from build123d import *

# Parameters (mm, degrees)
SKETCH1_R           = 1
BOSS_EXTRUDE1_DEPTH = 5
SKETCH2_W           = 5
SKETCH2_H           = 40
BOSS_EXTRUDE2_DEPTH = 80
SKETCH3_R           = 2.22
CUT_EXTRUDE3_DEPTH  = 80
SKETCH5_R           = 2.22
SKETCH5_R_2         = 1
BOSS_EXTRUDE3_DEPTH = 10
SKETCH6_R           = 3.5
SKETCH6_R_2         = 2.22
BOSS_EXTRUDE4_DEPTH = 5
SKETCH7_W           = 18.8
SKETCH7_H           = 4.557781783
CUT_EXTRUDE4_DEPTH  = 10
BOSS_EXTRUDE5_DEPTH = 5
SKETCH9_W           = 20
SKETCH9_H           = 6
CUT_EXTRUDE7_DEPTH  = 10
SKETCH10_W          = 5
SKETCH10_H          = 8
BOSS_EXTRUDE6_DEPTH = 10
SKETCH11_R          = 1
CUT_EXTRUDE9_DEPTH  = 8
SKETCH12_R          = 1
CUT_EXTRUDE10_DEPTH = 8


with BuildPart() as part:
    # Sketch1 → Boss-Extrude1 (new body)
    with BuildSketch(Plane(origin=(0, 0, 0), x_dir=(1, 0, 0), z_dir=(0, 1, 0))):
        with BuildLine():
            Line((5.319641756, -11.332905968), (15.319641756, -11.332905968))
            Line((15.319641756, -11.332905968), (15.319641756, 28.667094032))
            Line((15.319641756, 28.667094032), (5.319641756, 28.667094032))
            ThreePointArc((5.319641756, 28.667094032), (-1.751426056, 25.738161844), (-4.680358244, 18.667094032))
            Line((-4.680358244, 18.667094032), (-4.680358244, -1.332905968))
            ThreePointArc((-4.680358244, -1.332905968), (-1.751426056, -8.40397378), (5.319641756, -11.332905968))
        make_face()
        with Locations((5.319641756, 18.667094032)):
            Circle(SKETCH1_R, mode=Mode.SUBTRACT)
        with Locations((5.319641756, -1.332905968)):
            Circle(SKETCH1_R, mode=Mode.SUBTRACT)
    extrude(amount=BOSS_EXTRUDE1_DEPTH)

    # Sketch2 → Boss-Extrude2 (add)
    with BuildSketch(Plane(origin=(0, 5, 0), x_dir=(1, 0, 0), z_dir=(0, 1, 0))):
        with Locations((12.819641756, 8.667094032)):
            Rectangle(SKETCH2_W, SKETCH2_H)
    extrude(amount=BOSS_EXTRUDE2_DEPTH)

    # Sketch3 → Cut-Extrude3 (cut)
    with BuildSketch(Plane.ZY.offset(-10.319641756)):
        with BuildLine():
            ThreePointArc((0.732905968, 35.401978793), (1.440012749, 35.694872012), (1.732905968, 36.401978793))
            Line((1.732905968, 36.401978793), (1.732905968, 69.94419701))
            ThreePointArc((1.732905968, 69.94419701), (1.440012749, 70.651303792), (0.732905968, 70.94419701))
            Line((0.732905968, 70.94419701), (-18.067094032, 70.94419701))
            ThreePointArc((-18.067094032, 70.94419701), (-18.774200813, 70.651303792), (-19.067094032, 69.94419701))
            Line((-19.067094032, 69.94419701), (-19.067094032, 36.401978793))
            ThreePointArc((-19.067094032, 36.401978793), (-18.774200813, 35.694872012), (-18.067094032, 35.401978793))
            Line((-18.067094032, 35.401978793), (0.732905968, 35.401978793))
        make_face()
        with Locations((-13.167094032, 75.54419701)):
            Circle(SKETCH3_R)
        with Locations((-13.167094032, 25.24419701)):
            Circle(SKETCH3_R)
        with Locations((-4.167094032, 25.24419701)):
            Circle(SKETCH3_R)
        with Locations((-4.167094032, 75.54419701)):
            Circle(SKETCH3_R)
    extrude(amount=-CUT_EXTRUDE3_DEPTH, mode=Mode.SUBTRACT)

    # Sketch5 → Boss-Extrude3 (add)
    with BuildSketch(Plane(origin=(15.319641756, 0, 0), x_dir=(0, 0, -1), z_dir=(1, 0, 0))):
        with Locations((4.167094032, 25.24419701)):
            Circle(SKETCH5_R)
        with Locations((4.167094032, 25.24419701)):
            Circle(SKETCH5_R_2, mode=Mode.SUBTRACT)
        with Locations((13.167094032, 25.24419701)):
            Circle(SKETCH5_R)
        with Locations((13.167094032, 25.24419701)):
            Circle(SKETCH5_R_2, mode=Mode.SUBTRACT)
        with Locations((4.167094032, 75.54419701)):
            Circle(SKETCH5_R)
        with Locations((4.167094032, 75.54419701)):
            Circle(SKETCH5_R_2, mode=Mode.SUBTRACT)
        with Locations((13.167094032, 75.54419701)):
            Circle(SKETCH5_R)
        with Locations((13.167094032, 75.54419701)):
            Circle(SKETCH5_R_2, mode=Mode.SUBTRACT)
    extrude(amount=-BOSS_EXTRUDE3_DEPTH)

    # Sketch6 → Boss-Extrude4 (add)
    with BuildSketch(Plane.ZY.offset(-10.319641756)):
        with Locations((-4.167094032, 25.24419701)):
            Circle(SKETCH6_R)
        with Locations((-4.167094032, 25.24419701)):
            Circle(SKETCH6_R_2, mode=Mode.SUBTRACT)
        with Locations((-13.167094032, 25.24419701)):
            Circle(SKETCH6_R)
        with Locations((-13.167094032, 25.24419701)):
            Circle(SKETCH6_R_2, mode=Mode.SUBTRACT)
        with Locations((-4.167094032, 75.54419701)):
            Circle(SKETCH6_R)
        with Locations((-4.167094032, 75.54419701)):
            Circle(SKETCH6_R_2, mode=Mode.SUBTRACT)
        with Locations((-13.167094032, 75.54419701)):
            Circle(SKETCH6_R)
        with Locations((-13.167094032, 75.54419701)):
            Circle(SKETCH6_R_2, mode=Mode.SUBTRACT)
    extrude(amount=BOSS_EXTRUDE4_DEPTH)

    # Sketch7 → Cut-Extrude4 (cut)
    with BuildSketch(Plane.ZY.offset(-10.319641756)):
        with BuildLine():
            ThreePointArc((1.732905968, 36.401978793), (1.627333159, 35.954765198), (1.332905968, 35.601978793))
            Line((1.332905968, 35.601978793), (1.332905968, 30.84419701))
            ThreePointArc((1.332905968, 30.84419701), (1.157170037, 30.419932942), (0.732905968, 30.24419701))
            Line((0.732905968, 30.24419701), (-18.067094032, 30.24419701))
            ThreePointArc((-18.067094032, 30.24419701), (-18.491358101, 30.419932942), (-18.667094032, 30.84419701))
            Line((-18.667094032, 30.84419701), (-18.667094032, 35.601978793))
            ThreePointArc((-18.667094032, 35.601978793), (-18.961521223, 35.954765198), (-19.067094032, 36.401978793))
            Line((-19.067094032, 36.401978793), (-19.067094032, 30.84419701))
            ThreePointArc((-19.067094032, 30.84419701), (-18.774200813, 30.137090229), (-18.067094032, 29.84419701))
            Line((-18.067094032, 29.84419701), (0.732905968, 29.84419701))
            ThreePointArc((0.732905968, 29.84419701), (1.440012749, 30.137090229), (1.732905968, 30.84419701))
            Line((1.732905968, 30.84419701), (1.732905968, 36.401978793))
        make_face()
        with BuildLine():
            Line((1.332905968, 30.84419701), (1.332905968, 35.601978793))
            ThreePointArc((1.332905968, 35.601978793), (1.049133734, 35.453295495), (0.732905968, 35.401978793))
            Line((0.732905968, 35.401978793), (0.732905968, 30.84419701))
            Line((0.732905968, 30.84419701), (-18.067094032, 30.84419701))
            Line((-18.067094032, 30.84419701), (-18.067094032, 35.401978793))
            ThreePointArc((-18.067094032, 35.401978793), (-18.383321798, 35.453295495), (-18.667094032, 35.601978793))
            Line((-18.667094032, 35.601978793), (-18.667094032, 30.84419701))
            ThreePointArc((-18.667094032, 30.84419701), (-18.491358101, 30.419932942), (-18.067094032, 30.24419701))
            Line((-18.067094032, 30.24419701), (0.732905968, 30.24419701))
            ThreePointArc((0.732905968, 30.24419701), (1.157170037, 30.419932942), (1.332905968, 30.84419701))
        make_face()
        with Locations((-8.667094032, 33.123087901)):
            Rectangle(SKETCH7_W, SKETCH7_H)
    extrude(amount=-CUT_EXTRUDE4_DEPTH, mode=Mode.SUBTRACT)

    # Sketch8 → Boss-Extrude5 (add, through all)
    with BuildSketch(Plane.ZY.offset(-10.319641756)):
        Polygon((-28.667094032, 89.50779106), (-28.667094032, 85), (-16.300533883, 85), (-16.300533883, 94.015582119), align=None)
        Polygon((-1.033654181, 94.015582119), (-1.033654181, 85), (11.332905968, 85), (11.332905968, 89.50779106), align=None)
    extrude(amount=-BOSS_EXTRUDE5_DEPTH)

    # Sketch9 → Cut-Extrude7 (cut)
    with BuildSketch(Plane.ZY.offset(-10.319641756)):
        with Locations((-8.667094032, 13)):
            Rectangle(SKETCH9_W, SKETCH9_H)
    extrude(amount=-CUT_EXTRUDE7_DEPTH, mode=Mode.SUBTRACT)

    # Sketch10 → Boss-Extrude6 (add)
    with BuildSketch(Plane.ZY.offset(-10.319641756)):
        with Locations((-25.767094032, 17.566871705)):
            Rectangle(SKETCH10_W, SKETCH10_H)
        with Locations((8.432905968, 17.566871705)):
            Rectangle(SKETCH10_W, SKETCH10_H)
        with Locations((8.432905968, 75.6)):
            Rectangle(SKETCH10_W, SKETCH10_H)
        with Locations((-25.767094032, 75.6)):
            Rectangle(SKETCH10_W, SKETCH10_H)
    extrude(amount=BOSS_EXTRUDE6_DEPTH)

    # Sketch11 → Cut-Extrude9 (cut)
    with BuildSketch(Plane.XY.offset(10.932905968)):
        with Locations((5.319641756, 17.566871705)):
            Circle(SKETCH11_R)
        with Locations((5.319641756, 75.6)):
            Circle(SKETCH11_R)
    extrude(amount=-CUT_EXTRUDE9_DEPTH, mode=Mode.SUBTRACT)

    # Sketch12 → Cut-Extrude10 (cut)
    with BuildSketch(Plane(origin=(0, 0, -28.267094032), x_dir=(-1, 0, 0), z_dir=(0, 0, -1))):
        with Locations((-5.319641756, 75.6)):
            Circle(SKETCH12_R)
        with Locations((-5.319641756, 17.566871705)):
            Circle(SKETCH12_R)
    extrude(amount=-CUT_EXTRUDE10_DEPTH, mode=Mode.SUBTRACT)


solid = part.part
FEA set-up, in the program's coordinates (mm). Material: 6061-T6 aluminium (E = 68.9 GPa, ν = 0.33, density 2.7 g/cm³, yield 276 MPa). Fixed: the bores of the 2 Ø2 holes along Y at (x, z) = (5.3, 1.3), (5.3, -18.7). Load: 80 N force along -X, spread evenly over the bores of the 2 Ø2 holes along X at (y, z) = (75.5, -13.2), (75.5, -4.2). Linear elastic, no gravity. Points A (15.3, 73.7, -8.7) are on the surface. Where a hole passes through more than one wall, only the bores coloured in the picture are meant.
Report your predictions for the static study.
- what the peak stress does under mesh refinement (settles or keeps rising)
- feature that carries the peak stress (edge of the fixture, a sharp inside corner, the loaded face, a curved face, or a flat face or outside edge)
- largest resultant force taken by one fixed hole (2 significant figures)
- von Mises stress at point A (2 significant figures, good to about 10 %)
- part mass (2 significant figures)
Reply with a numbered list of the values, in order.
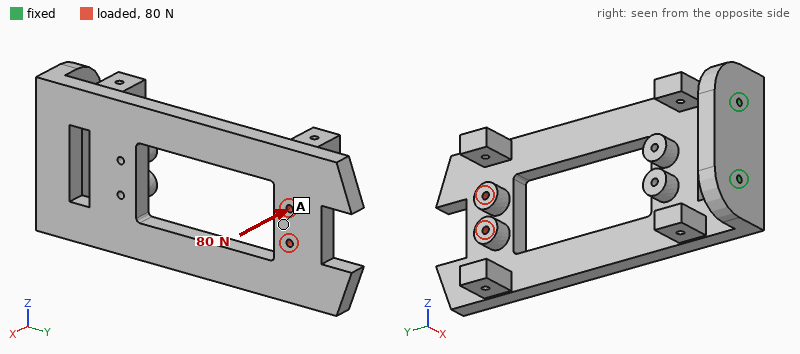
1. keeps rising
2. edge of the fixture
3. 40 N
4. 6.8 MPa
5. 48 g
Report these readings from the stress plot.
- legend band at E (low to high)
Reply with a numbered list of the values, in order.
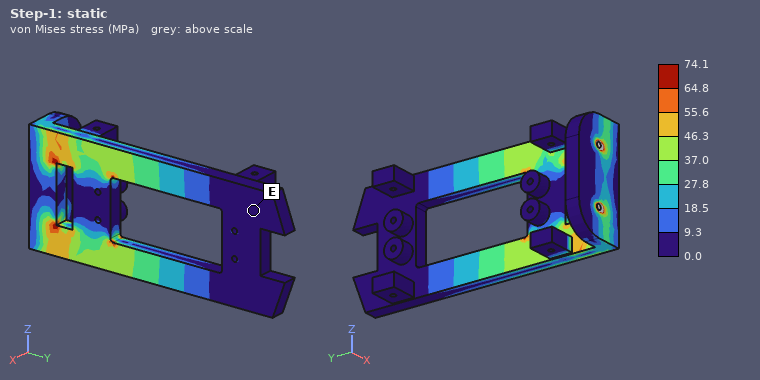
1. 0.0 to 9.3 MPa
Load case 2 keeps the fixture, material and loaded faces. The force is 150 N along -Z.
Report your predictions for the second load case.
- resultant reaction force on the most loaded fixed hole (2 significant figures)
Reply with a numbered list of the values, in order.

1. 460 N
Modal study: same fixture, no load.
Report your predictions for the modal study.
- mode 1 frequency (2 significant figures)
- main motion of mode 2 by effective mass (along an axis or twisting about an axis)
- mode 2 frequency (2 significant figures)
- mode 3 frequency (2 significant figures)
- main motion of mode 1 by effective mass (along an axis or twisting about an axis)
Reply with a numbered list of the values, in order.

1. 380 Hz
2. along Z
3. 1300 Hz
4. 1700 Hz
5. along X
